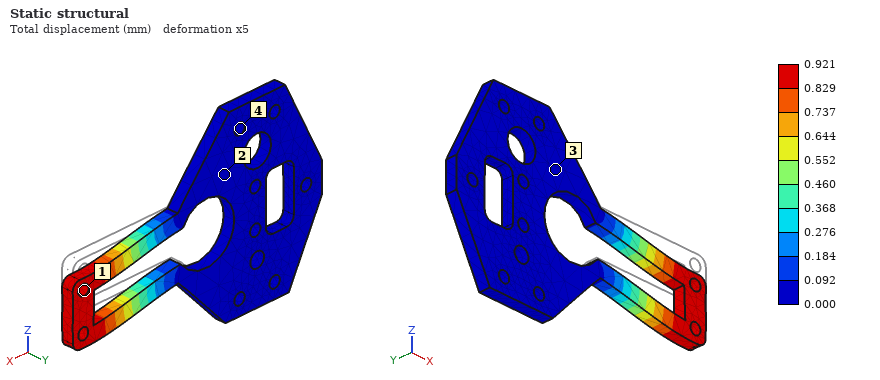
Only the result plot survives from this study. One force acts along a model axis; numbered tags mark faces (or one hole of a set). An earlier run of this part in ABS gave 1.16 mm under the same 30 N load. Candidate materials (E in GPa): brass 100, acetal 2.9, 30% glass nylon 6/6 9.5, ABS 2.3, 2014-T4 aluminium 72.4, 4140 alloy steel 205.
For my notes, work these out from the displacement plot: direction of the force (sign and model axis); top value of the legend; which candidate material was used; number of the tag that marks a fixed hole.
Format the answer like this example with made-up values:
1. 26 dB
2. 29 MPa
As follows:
1. -Z
2. 0.921 mm
3. acetal
4. 4
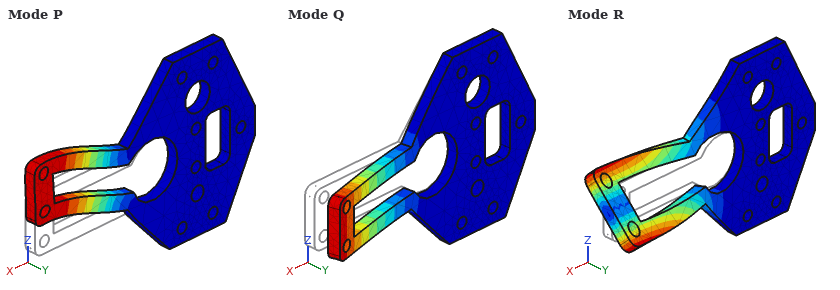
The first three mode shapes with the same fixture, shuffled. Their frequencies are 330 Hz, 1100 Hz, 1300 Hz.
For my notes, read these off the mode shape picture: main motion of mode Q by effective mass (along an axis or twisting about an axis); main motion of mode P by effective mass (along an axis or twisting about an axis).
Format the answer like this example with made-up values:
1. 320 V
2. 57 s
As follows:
1. along Y
2. along Z
